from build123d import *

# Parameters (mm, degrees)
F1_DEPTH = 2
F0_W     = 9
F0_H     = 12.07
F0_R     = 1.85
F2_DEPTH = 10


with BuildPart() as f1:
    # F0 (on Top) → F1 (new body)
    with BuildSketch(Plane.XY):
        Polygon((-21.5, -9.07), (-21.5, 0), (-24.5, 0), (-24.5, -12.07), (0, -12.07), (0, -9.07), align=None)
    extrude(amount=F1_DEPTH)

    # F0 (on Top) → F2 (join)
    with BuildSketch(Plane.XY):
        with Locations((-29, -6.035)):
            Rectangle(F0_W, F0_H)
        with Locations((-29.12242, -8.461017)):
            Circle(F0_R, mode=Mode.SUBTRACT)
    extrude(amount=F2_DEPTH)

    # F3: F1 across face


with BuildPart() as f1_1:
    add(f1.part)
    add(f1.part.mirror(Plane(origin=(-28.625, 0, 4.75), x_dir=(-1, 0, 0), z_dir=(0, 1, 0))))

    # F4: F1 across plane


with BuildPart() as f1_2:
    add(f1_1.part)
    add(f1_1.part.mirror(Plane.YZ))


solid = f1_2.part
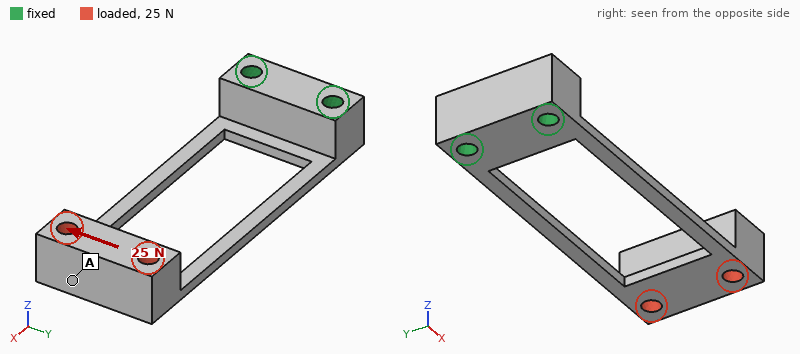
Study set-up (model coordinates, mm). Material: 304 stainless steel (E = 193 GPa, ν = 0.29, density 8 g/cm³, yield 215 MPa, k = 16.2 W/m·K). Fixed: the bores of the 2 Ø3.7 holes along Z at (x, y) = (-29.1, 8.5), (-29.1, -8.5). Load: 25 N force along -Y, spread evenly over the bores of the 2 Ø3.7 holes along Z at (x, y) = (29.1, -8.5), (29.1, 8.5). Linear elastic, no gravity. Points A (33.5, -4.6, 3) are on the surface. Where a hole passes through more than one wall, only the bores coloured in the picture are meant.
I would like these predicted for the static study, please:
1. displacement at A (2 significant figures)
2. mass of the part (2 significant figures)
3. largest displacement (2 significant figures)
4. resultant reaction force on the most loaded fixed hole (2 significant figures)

0.14 mm
38 g
0.17 mm
70 N
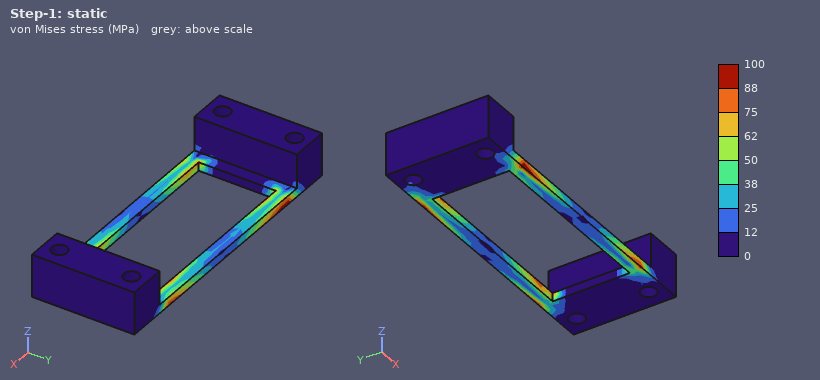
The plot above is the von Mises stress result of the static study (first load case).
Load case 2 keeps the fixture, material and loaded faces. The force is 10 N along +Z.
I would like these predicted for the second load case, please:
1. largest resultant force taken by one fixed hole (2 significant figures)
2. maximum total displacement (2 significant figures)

5.2 N
0.75 mm
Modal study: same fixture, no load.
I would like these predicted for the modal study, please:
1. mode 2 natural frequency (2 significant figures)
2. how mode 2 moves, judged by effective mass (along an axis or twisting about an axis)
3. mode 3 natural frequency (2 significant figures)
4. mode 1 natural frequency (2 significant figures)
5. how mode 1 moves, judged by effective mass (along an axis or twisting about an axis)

490 Hz
along Y
810 Hz
150 Hz
along Z
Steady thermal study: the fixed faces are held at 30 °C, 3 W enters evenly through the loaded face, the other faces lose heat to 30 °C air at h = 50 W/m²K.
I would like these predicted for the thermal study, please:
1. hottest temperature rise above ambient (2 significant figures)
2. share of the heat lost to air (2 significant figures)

45 K
99 %
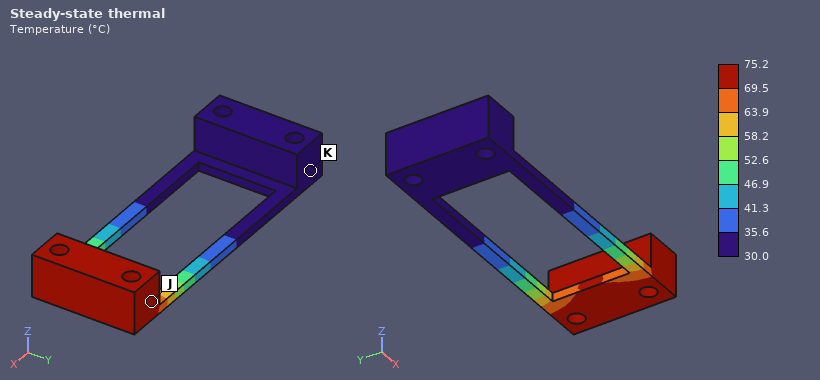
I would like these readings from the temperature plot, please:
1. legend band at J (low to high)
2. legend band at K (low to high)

69.5 to 75.2 °C
30.0 to 35.6 °C
